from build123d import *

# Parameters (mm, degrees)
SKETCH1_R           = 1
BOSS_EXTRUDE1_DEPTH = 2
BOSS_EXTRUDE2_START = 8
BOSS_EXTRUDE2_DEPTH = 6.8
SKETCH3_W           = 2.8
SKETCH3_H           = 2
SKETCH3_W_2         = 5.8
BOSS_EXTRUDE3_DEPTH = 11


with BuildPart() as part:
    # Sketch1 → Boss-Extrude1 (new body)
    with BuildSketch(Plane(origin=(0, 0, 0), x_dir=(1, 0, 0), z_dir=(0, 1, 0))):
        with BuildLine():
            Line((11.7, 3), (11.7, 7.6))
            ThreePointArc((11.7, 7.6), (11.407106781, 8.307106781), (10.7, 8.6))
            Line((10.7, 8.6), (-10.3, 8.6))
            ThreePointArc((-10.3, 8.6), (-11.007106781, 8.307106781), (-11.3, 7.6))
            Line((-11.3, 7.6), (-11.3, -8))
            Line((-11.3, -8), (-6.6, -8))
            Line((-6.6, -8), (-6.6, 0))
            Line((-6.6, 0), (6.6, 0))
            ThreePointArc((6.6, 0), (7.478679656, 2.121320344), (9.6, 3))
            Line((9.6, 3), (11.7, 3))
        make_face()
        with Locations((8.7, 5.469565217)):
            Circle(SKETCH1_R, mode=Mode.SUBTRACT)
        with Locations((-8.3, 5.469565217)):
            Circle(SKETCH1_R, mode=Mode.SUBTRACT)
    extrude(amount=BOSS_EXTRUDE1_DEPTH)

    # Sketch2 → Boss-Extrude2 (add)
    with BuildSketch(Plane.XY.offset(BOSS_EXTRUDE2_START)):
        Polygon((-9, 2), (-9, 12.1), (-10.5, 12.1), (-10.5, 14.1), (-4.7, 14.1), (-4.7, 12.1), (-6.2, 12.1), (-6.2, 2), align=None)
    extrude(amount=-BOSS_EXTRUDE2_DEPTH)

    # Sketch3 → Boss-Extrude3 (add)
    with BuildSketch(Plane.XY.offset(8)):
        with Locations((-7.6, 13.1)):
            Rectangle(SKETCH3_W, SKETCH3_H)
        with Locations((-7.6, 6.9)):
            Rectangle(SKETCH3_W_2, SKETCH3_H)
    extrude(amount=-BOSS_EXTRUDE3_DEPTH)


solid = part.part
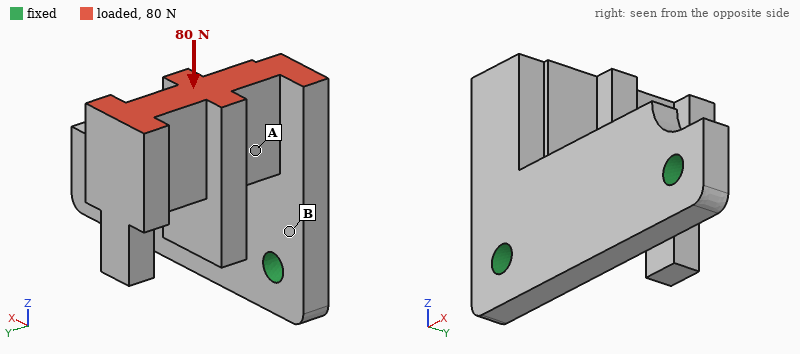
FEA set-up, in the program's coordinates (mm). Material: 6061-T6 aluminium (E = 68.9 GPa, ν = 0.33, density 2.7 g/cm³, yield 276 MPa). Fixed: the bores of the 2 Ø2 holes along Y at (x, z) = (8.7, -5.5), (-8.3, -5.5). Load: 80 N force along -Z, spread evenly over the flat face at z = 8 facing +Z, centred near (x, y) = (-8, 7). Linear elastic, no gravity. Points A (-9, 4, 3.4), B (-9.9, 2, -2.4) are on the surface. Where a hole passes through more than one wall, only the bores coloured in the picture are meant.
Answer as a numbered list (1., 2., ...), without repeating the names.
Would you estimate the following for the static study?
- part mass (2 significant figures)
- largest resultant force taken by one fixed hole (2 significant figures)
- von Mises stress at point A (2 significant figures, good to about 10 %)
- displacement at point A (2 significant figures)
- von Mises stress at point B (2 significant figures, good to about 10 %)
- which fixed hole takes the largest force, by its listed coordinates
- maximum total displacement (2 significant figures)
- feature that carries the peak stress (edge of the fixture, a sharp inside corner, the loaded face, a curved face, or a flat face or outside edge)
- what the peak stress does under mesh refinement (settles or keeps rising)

1. 2.2 g
2. 77 N
3. 22 MPa
4. 0.075 mm
5. 120 MPa
6. (-8.3, -5.5)
7. 0.23 mm
8. a sharp inside corner
9. keeps rising
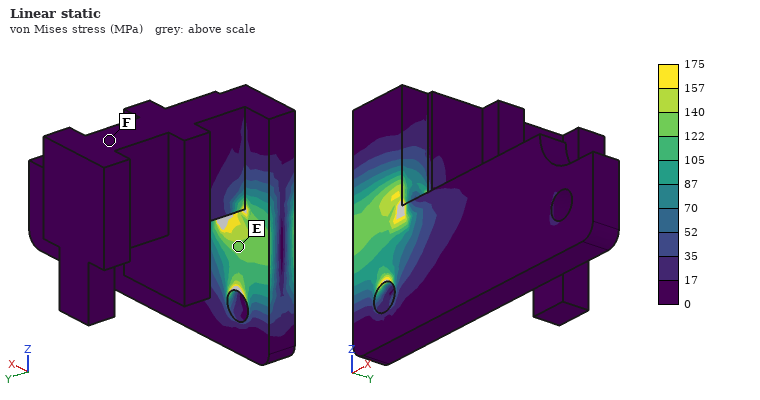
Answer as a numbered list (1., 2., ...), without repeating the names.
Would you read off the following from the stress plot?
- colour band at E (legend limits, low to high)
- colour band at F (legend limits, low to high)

1. 122 to 140 MPa
2. 0 to 17 MPa
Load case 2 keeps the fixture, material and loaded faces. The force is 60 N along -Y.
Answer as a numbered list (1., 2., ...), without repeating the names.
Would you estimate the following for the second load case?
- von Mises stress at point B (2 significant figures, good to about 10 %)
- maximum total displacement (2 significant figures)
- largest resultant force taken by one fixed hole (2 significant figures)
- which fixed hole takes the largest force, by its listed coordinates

1. 130 MPa
2. 0.25 mm
3. 64 N
4. (-8.3, -5.5)
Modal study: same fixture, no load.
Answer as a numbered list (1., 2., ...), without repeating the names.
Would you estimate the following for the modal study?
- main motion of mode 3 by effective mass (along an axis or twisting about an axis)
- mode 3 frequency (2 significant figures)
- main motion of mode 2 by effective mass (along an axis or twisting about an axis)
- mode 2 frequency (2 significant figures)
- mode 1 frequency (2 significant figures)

1. along Y
2. 12 kHz
3. along X
4. 3500 Hz
5. 2800 Hz
